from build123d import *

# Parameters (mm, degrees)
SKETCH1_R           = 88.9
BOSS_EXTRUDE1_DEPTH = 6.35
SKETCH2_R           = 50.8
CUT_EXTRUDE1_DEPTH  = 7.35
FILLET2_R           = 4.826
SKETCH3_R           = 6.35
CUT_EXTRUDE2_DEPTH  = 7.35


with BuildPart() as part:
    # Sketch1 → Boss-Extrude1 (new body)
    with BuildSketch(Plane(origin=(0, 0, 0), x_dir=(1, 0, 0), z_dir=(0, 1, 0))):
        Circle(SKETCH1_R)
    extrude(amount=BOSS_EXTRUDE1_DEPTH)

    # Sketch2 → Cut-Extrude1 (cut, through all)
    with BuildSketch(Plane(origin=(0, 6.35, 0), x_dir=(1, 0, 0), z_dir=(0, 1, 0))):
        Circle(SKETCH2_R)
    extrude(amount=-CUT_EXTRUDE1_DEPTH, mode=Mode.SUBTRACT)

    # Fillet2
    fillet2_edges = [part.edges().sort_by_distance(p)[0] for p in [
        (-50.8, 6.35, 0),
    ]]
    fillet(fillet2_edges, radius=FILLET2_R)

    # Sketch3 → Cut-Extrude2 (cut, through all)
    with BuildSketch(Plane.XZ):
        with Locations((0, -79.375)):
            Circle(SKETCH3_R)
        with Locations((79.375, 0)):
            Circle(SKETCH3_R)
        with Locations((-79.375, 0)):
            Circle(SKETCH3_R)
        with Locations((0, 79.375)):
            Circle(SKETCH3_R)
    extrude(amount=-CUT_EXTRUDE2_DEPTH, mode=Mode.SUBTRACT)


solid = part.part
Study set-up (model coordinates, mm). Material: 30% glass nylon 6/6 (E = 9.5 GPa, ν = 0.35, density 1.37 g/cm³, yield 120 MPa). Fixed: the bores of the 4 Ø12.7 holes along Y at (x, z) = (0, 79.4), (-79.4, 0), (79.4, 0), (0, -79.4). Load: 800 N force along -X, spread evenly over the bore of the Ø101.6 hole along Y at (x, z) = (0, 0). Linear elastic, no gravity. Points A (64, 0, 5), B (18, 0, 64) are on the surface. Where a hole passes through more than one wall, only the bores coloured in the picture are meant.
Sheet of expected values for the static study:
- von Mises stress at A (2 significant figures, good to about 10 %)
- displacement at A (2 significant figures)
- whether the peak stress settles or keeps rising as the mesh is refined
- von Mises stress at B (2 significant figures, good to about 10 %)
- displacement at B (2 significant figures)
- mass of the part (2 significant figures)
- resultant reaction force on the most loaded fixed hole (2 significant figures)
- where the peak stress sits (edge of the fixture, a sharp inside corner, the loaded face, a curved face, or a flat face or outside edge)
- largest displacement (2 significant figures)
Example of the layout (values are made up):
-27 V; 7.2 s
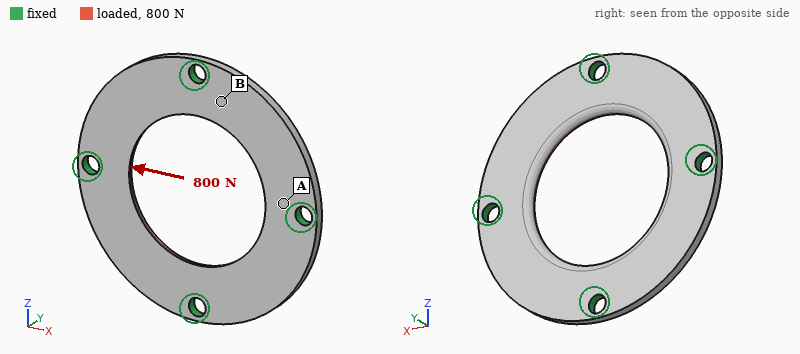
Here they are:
1.6 MPa; 2.3 µm; keeps rising; 0.68 MPa; 3.9 µm; 140 g; 220 N; edge of the fixture; 12 µm
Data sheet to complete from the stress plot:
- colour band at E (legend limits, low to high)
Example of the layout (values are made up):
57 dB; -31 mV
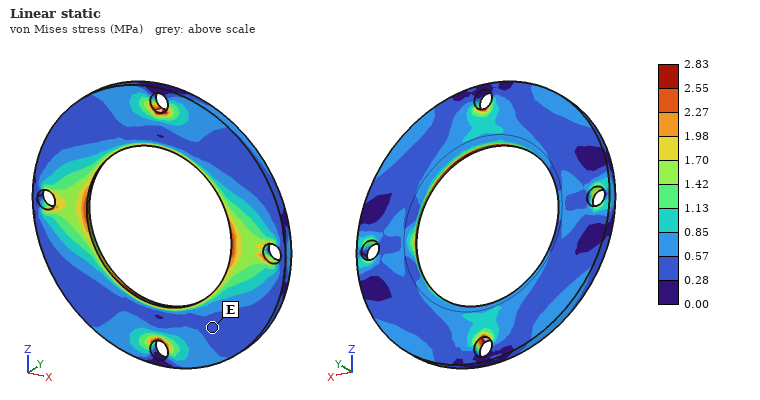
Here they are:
0.28 to 0.57 MPa
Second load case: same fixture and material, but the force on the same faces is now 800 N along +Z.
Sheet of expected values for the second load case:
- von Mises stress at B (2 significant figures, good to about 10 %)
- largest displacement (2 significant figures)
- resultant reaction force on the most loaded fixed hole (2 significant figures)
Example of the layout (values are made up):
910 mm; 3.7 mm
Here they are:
1.2 MPa; 12 µm; 220 N
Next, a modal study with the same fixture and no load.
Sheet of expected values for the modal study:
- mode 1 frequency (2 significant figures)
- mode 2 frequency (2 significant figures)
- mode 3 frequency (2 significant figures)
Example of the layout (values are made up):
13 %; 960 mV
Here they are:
1300 Hz; 1300 Hz; 1300 Hz
